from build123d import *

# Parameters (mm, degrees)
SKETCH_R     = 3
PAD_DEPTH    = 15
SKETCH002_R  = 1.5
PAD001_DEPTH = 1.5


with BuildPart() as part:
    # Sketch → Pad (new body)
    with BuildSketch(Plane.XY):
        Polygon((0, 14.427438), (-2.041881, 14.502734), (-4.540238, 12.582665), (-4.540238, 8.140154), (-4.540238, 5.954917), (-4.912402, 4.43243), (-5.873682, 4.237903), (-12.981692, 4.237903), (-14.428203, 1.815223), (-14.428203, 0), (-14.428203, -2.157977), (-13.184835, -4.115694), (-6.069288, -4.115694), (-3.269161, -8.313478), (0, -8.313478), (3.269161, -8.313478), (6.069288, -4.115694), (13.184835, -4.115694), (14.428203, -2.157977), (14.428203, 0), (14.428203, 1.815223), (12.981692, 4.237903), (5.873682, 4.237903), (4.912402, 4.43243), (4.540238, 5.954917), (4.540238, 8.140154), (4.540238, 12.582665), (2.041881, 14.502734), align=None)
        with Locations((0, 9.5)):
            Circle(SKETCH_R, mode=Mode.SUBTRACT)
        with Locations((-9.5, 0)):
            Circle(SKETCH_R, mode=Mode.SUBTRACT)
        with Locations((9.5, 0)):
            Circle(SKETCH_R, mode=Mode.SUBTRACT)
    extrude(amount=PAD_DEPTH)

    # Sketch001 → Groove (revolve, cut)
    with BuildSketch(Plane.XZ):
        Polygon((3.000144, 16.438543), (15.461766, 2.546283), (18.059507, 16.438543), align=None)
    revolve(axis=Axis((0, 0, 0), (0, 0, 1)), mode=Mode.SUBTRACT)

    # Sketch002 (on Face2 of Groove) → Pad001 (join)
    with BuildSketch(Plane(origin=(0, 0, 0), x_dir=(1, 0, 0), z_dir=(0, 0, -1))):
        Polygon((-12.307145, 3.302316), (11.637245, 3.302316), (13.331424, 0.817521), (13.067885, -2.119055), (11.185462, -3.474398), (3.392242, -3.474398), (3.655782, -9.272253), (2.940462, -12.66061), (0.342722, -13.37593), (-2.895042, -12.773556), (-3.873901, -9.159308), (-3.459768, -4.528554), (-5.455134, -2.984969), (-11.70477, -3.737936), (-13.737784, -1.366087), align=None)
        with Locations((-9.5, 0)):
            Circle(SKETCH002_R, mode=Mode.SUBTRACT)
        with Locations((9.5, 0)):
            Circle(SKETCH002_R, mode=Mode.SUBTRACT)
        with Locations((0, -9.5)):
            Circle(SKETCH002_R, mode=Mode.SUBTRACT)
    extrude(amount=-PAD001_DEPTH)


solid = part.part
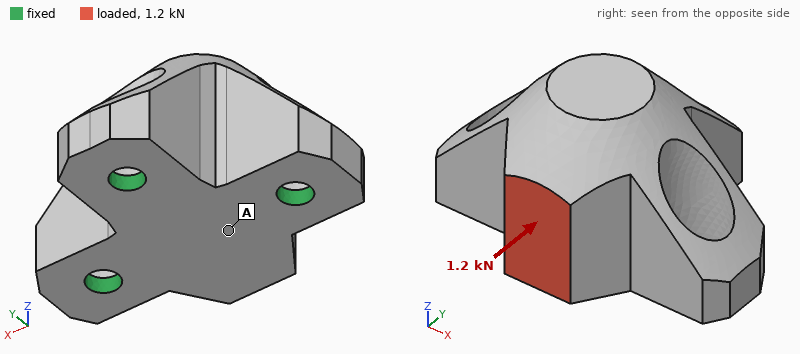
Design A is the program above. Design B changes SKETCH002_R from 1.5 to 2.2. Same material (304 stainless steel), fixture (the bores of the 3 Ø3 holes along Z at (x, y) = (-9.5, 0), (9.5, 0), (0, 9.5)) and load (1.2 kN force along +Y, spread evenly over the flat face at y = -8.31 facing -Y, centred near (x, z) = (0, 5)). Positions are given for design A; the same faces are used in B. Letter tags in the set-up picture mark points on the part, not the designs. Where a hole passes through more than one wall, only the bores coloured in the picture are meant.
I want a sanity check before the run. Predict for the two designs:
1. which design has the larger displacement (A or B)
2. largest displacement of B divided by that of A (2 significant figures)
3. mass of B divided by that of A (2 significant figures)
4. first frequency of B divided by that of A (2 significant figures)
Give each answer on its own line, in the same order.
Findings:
A
0.61
0.99
1.3
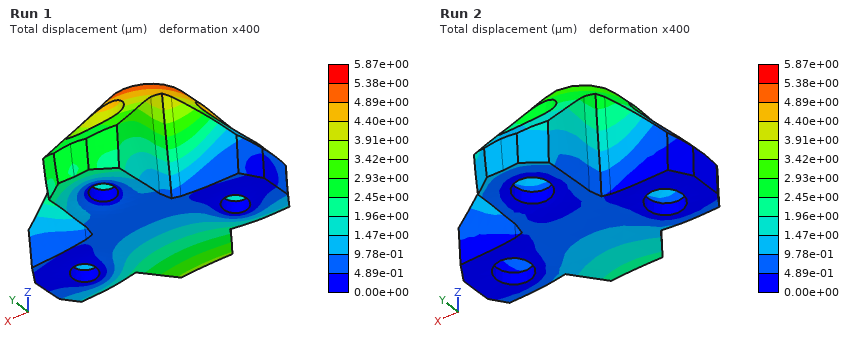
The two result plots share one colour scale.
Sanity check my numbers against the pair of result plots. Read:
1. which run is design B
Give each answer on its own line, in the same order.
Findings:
Run 2
